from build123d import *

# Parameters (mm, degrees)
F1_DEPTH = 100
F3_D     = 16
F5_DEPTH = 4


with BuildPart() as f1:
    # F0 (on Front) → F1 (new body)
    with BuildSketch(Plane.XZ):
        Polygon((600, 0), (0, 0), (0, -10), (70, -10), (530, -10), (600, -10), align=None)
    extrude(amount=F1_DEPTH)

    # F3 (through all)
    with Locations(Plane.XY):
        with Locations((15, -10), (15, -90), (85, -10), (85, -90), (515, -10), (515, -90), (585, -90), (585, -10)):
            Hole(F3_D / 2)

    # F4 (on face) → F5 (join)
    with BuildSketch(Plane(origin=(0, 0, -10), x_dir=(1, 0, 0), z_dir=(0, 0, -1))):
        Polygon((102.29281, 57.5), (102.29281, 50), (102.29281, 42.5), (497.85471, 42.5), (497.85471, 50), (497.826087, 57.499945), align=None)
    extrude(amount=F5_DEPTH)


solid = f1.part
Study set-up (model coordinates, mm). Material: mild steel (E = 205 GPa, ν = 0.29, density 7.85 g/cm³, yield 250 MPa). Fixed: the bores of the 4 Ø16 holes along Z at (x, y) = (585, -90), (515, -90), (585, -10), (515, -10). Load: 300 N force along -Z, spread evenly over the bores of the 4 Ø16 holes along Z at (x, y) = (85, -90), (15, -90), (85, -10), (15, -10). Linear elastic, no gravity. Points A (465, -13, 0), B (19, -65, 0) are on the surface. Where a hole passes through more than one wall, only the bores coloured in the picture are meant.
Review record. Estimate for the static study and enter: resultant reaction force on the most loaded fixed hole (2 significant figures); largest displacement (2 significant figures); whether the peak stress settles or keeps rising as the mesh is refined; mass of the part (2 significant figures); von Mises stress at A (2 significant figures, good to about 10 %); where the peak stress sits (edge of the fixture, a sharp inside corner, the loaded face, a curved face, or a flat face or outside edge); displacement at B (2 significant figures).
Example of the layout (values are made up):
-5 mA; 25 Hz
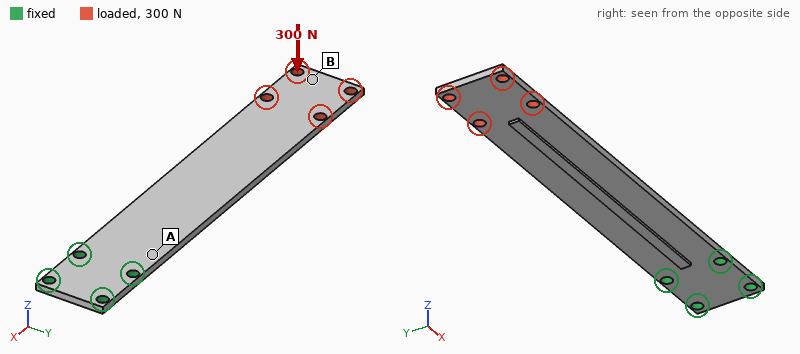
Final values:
400 N; 5.3 mm; keeps rising; 4.8 kg; 61 MPa; edge of the fixture; 5.0 mm
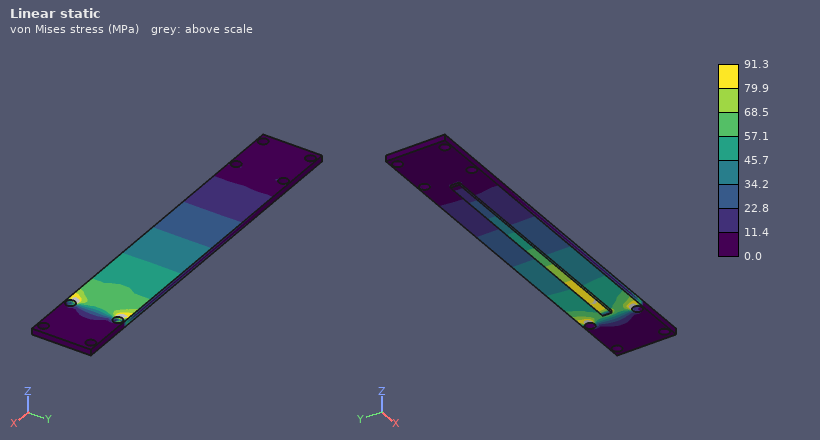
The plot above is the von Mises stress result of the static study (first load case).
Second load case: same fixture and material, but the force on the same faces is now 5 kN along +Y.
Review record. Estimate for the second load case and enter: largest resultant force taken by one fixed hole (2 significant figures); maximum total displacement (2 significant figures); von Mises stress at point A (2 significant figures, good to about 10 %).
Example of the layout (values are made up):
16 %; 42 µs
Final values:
28 kN; 1.2 mm; 91 MPa
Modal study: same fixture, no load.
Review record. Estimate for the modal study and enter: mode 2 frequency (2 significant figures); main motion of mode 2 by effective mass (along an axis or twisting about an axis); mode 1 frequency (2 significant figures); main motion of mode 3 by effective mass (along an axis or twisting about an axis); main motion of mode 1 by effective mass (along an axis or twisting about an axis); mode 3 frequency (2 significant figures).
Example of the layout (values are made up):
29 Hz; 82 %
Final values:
220 Hz; along Z; 36 Hz; along Y; along Z; 310 Hz
